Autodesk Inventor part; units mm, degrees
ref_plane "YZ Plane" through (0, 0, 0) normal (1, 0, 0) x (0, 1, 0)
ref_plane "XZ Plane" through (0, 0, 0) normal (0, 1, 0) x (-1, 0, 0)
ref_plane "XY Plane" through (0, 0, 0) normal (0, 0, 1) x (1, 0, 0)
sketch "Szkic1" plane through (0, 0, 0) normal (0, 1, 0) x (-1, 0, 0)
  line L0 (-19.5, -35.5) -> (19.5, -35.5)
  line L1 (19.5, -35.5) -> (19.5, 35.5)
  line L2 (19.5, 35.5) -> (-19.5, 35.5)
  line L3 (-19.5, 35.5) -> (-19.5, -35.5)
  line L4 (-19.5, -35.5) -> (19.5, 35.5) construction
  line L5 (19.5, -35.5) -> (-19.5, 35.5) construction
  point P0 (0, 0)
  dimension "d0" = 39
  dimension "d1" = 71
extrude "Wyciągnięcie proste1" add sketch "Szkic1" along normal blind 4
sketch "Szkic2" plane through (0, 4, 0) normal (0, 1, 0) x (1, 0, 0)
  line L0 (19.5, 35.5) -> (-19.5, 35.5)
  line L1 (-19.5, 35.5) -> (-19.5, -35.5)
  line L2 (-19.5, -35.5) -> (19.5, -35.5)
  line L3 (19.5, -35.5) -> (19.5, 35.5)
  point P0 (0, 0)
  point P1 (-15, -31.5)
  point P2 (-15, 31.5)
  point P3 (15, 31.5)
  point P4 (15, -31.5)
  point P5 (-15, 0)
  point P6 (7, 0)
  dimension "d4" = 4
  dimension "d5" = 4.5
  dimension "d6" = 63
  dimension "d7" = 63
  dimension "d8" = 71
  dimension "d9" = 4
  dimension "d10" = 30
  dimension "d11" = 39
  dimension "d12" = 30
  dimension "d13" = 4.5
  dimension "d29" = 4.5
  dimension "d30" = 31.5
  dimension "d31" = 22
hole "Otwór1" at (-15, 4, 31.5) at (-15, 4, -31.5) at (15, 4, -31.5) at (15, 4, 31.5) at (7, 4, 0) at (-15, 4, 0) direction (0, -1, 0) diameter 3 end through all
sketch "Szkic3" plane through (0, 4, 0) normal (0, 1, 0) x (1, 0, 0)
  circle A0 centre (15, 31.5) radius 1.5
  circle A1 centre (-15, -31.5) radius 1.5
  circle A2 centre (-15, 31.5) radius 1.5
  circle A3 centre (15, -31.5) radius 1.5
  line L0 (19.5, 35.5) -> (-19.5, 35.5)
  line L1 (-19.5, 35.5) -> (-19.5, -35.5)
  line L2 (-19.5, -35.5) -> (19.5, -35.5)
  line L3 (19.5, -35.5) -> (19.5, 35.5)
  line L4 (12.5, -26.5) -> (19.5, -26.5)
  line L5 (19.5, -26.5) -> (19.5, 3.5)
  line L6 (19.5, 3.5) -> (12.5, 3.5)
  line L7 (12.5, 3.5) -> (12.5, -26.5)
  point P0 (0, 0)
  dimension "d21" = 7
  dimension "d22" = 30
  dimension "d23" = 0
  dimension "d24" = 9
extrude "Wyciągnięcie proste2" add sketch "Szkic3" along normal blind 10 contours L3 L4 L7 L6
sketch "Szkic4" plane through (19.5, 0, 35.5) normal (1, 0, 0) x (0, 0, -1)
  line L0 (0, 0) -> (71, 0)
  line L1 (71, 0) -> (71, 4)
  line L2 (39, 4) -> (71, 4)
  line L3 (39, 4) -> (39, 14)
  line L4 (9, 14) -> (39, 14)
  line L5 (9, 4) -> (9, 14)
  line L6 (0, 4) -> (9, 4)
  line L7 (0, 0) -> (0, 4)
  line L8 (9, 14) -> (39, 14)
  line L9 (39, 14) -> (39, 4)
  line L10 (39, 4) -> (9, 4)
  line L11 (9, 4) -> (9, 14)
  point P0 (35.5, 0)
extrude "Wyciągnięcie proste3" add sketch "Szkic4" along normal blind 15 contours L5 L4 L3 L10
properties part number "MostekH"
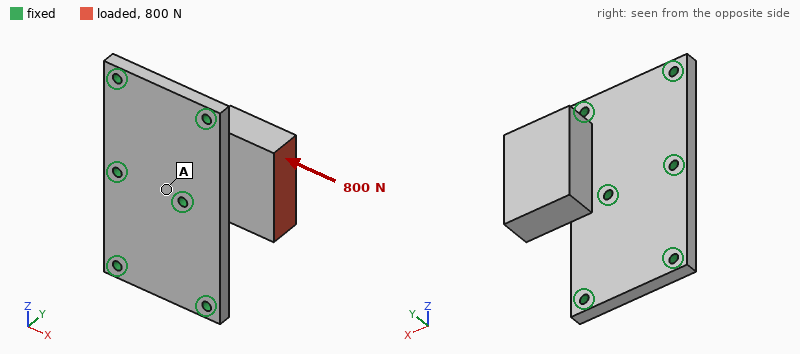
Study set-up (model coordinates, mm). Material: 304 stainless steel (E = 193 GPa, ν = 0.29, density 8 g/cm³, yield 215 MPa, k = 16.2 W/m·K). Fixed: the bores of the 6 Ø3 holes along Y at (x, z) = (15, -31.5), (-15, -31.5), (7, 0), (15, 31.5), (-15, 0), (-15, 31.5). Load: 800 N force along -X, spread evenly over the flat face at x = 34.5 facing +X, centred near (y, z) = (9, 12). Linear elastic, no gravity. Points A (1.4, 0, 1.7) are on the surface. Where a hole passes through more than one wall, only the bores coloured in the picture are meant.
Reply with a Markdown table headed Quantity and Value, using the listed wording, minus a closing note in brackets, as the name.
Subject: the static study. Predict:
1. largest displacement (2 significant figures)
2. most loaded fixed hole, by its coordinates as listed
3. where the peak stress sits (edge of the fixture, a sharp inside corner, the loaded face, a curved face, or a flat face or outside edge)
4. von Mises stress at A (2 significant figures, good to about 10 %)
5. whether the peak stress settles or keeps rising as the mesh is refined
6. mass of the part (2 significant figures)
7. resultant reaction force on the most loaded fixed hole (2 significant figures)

| Quantity | Value |
|---|---|
| largest displacement | 22 µm |
| most loaded fixed hole, by its coordinates as listed | (7, 0) |
| where the peak stress sits | edge of the fixture |
| von Mises stress at A | 8.0 MPa |
| whether the peak stress settles or keeps rising as the mesh is refined | keeps rising |
| mass of the part | 140 g |
| resultant reaction force on the most loaded fixed hole | 390 N |
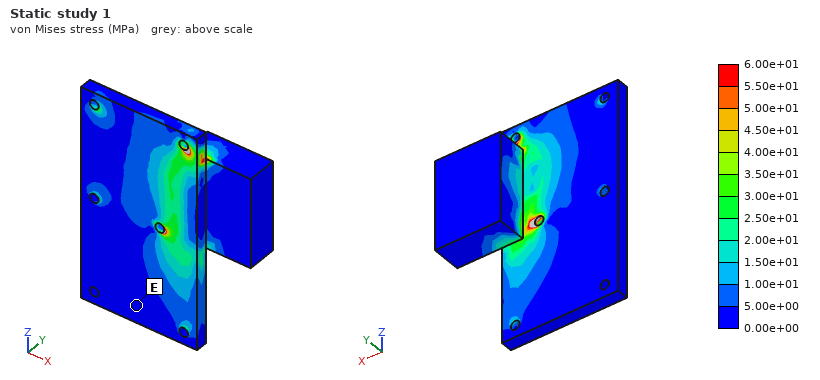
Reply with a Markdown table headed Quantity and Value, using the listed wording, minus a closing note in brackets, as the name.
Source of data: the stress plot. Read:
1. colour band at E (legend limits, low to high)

| Quantity | Value |
|---|---|
| colour band at E | 0.00e+00 to 5.00e+00 MPa |
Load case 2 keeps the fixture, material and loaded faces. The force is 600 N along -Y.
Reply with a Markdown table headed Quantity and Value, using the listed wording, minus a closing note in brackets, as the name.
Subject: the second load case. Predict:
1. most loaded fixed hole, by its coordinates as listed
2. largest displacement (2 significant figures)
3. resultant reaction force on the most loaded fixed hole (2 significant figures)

| Quantity | Value |
|---|---|
| most loaded fixed hole, by its coordinates as listed | (15, 31.5) |
| largest displacement | 59 µm |
| resultant reaction force on the most loaded fixed hole | 540 N |
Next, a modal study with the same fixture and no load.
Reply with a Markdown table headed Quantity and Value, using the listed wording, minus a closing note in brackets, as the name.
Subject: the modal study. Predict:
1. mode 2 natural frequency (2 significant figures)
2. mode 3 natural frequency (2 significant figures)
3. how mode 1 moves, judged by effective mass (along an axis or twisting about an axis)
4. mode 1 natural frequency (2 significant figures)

| Quantity | Value |
|---|---|
| mode 2 natural frequency | 14 kHz |
| mode 3 natural frequency | 14 kHz |
| how mode 1 moves, judged by effective mass | along Y |
| mode 1 natural frequency | 3600 Hz |
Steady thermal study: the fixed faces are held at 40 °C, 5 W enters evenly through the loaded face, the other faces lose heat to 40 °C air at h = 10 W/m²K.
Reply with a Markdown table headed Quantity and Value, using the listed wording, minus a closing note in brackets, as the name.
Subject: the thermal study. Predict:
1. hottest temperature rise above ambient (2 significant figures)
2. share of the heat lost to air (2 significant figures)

| Quantity | Value |
|---|---|
| hottest temperature rise above ambient | 39 K |
| share of the heat lost to air | 15 % |
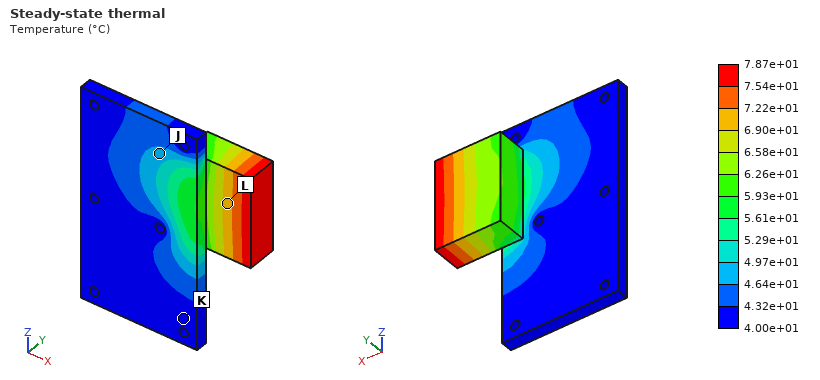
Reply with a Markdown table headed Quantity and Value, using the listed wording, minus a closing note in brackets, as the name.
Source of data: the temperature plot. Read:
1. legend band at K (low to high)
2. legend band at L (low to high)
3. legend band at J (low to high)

| Quantity | Value |
|---|---|
| legend band at K | 4.00e+01 to 4.32e+01 °C |
| legend band at L | 6.90e+01 to 7.22e+01 °C |
| legend band at J | 4.64e+01 to 4.97e+01 °C |
